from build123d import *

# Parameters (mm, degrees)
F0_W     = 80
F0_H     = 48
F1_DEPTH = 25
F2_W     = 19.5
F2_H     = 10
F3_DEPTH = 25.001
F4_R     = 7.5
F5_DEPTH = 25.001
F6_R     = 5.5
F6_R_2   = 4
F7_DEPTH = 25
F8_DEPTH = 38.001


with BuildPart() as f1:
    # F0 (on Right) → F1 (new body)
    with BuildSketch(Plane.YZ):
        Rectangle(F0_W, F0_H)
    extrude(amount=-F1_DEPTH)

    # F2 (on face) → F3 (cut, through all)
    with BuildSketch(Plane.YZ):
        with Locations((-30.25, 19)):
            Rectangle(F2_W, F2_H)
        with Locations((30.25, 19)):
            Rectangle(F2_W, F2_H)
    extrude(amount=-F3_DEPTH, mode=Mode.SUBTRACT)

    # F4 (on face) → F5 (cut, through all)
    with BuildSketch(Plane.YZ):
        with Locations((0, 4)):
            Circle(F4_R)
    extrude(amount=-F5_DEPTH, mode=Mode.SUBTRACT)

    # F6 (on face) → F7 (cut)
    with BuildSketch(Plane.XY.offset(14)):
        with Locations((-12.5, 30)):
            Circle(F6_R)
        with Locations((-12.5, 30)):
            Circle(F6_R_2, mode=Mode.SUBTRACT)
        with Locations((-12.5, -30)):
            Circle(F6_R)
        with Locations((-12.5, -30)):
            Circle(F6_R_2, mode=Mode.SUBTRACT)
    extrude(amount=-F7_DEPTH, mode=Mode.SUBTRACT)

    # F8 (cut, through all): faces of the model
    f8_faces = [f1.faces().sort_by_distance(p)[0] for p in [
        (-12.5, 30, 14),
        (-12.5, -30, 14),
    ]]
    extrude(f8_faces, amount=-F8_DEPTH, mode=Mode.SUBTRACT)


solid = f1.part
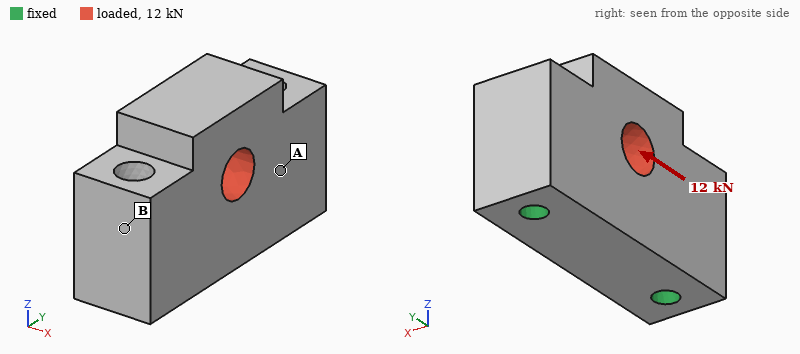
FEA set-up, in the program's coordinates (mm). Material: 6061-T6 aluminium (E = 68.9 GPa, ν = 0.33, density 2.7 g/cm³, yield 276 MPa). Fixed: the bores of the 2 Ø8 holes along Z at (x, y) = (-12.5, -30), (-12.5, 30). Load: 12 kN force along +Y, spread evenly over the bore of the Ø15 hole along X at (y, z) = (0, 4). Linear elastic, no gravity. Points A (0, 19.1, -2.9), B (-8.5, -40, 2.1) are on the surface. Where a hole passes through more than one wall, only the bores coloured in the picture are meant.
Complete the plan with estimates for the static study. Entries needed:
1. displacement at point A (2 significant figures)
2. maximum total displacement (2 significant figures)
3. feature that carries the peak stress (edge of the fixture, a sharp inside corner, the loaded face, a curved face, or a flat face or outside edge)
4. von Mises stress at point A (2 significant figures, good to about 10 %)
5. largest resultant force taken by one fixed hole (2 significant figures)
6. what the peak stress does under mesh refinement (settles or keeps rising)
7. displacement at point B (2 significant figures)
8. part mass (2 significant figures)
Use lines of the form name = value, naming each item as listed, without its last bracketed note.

displacement at point A = 6.6 µm
maximum total displacement = 14 µm
feature that carries the peak stress = edge of the fixture
von Mises stress at point A = 13 MPa
largest resultant force taken by one fixed hole = 7.1 kN
what the peak stress does under mesh refinement = keeps rising
displacement at point B = 9.2 µm
part mass = 200 g
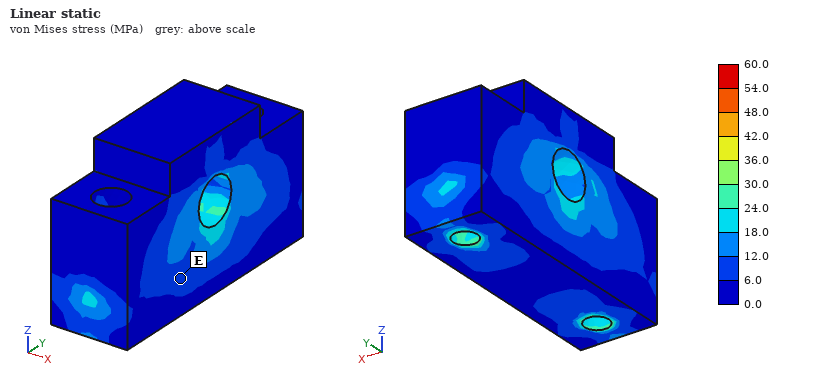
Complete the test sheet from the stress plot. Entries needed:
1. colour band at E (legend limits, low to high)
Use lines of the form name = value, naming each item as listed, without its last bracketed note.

colour band at E = 6.0 to 12.0 MPa
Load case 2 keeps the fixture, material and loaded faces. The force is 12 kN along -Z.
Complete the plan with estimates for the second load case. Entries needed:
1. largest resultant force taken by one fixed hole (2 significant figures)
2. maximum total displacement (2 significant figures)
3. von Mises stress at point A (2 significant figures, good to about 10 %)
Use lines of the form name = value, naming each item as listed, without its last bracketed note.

largest resultant force taken by one fixed hole = 6.6 kN
maximum total displacement = 12 µm
von Mises stress at point A = 12 MPa
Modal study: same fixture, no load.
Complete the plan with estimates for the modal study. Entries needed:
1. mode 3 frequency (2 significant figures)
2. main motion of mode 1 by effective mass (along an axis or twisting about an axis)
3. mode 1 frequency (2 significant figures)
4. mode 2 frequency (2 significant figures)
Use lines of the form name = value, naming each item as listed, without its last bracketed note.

mode 3 frequency = 14 kHz
main motion of mode 1 by effective mass = along X
mode 1 frequency = 5700 Hz
mode 2 frequency = 14 kHz
